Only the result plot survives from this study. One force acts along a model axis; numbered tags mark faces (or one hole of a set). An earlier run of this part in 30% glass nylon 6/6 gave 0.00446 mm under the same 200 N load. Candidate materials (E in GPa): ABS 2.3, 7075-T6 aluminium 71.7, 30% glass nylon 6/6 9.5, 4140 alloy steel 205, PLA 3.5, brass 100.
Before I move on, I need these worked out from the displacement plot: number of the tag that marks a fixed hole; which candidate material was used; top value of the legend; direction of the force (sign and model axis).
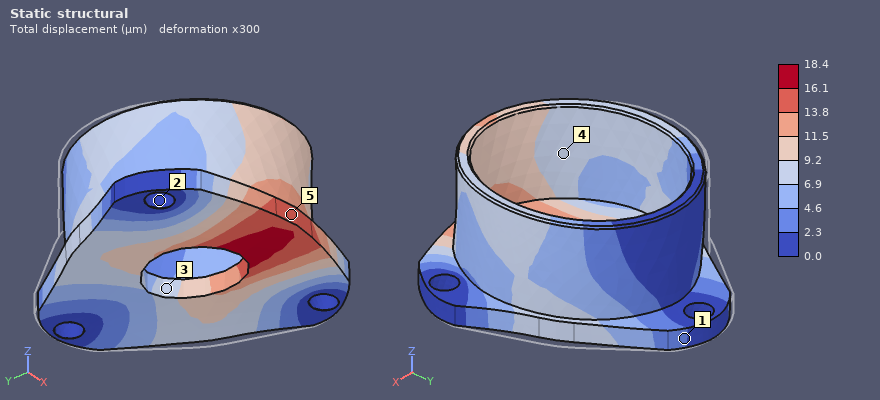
2
ABS
18.4 µm
-Y
